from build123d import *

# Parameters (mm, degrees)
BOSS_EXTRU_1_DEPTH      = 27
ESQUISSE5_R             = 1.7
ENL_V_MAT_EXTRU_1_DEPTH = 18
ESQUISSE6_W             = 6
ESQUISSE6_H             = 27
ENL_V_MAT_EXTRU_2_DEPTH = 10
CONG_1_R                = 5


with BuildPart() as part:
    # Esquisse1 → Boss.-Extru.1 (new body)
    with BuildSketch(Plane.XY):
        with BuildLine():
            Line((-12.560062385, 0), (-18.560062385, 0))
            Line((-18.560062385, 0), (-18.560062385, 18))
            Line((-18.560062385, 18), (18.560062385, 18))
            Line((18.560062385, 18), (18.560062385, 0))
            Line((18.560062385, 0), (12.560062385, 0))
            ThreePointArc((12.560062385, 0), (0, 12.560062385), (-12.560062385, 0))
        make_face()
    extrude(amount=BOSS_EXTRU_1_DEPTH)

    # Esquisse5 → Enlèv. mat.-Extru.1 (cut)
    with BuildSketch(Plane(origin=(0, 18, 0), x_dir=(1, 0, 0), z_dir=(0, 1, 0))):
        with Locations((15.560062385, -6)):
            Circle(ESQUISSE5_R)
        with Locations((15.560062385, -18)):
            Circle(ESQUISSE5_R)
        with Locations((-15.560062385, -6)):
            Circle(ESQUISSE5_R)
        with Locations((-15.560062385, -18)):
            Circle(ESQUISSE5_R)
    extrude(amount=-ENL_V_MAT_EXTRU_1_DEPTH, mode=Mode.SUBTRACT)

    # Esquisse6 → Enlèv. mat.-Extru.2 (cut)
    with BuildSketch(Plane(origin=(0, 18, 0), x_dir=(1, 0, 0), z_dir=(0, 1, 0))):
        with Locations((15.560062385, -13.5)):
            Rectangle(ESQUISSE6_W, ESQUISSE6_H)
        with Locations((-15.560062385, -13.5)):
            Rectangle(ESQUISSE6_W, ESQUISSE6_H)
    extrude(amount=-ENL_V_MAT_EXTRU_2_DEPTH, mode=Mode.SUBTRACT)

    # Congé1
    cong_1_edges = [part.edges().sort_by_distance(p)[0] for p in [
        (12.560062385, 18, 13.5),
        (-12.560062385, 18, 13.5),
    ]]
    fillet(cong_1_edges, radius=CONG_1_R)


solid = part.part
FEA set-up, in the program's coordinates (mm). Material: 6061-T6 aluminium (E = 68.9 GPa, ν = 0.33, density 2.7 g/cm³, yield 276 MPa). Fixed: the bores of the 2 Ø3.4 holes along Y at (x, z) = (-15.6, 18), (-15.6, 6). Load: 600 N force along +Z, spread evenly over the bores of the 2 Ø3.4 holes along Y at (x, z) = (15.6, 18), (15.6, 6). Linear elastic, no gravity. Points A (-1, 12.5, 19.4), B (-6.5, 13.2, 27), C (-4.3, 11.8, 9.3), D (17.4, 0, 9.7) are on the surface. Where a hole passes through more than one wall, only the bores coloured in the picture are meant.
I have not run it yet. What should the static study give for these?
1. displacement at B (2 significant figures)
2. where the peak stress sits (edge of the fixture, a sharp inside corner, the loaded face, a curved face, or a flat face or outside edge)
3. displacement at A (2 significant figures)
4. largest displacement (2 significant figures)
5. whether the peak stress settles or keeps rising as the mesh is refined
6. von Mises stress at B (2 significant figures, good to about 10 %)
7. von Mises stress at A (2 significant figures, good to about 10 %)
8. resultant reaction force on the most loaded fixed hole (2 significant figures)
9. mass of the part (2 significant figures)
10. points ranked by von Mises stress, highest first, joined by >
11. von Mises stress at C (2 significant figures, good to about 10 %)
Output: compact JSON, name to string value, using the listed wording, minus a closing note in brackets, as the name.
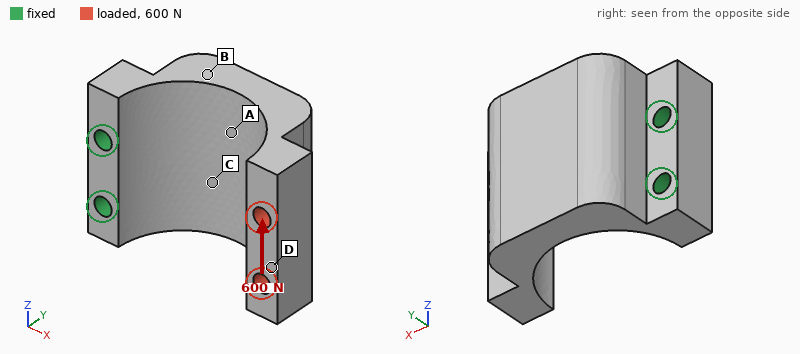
{"displacement at B": "0.054 mm", "where the peak stress sits": "edge of the fixture", "displacement at A": "0.045 mm", "largest displacement": "0.18 mm", "whether the peak stress settles or keeps rising as the mesh is refined": "keeps rising", "von Mises stress at B": "30 MPa", "von Mises stress at A": "63 MPa", "resultant reaction force on the most loaded fixed hole": "1.2 kN", "mass of the part": "20 g", "points ranked by von Mises stress, highest first, joined by >": "C > A > B > D", "von Mises stress at C": "85 MPa"}
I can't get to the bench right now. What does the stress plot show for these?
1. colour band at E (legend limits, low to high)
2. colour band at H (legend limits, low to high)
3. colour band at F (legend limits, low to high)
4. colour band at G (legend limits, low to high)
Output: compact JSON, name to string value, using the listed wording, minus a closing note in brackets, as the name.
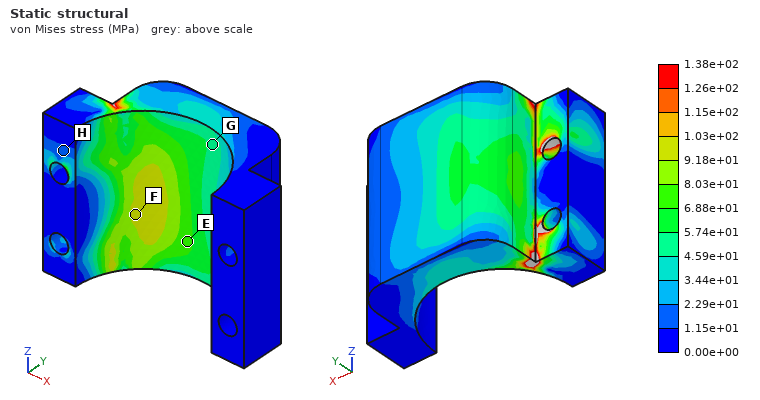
{"colour band at E": "6.88e+01 to 8.03e+01 MPa", "colour band at H": "1.15e+01 to 2.29e+01 MPa", "colour band at F": "9.18e+01 to 1.03e+02 MPa", "colour band at G": "4.59e+01 to 5.74e+01 MPa"}
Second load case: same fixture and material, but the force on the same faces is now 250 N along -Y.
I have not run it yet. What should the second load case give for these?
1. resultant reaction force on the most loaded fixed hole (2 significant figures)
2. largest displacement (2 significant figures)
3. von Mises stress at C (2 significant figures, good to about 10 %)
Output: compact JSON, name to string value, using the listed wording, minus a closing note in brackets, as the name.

{"resultant reaction force on the most loaded fixed hole": "140 N", "largest displacement": "0.36 mm", "von Mises stress at C": "32 MPa"}
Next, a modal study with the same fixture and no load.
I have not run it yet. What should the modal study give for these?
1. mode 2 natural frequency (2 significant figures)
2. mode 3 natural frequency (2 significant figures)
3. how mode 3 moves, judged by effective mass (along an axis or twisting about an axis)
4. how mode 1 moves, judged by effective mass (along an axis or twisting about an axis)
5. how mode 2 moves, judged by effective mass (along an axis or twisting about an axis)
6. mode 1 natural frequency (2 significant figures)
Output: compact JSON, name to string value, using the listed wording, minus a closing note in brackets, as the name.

{"mode 2 natural frequency": "4200 Hz", "mode 3 natural frequency": "7700 Hz", "how mode 3 moves, judged by effective mass": "along X", "how mode 1 moves, judged by effective mass": "along Y", "how mode 2 moves, judged by effective mass": "along Z", "mode 1 natural frequency": "1700 Hz"}
